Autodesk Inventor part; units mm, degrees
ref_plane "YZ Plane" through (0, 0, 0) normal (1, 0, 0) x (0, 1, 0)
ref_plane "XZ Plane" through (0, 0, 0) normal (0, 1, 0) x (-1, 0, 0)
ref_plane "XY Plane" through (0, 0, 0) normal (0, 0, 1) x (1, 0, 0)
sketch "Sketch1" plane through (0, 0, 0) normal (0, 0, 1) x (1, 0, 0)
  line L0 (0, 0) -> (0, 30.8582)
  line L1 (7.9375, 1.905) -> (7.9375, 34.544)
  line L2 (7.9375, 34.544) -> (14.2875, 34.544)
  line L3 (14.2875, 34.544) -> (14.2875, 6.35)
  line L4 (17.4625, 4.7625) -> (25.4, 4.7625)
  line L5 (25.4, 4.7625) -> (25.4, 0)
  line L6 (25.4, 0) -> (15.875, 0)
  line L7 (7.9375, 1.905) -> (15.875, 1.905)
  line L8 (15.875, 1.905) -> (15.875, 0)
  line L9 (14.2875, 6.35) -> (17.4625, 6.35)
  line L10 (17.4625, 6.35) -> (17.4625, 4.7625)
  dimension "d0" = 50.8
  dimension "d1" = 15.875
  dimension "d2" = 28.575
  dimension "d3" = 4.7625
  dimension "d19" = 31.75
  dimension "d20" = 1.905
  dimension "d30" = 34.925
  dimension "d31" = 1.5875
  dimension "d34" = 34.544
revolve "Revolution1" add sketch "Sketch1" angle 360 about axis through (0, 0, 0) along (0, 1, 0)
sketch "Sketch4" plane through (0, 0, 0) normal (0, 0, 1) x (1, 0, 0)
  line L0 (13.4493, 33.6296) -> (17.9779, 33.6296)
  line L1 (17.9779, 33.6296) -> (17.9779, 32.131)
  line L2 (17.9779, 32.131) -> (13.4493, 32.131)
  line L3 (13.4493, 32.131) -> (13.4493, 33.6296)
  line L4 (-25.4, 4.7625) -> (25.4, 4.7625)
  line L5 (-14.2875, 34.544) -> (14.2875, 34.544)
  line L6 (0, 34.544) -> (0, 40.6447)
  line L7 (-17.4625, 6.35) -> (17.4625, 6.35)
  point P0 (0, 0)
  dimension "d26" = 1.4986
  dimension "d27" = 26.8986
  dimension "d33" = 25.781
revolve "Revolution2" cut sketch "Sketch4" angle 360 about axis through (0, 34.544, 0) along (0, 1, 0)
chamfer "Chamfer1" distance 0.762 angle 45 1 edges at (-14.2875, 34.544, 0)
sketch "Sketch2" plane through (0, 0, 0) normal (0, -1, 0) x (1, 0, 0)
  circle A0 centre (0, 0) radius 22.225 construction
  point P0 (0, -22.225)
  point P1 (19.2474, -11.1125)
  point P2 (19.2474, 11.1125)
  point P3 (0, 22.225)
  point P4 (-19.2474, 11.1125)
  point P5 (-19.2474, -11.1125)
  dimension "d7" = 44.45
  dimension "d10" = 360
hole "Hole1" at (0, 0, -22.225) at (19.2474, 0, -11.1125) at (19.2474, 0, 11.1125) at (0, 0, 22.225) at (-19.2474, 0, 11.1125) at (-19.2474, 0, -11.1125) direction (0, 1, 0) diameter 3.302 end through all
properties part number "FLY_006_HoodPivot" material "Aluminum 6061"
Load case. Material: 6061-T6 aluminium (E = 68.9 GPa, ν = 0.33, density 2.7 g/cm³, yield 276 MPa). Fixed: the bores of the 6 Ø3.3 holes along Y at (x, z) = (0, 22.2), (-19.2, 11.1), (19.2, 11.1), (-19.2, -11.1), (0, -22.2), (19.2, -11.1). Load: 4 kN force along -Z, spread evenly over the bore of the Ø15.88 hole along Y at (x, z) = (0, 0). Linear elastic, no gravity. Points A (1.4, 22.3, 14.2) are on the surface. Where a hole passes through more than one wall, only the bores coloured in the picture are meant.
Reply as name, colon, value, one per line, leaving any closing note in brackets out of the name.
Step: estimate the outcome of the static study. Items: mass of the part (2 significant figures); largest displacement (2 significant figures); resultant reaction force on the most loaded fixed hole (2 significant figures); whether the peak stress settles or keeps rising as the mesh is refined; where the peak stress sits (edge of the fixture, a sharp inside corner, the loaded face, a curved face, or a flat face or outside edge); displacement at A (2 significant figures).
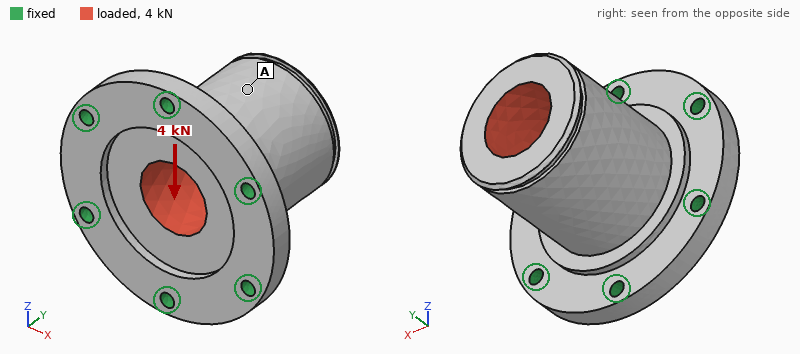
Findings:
mass of the part: 56 g
largest displacement: 39 µm
resultant reaction force on the most loaded fixed hole: 1.5 kN
whether the peak stress settles or keeps rising as the mesh is refined: keeps rising
where the peak stress sits: edge of the fixture
displacement at A: 27 µm
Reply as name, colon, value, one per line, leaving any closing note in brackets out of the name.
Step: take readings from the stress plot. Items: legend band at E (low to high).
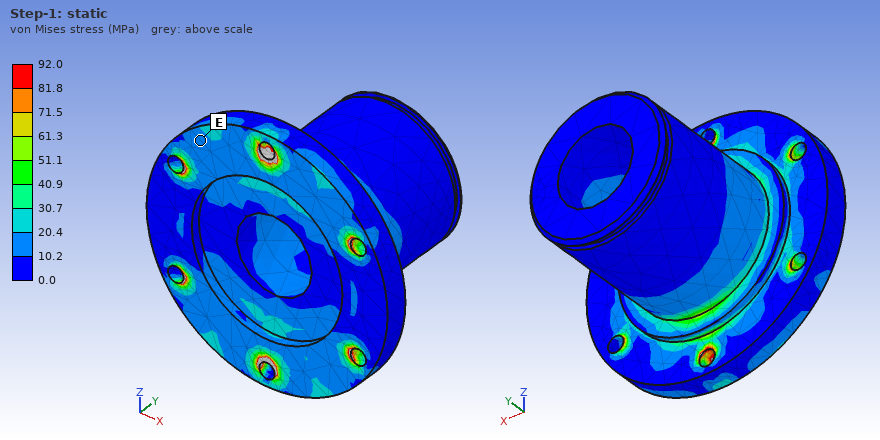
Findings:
legend band at E: 10.2 to 20.4 MPa
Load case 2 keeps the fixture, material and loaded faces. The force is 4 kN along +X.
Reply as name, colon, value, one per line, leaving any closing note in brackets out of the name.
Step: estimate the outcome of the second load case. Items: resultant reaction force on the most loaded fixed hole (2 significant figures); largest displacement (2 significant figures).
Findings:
resultant reaction force on the most loaded fixed hole: 1.3 kN
largest displacement: 39 µm
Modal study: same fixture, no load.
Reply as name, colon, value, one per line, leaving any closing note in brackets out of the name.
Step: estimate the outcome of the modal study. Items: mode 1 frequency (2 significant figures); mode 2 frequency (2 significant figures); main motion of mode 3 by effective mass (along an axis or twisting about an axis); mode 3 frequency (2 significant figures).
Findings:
mode 1 frequency: 9500 Hz
mode 2 frequency: 9500 Hz
main motion of mode 3 by effective mass: along Y
mode 3 frequency: 15 kHz
